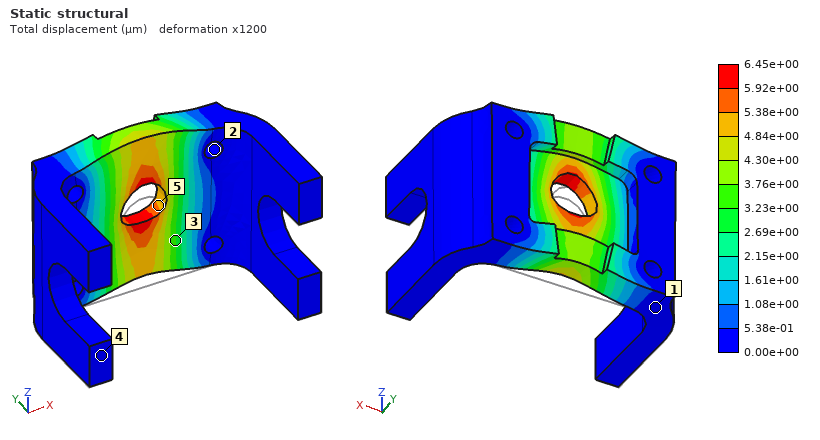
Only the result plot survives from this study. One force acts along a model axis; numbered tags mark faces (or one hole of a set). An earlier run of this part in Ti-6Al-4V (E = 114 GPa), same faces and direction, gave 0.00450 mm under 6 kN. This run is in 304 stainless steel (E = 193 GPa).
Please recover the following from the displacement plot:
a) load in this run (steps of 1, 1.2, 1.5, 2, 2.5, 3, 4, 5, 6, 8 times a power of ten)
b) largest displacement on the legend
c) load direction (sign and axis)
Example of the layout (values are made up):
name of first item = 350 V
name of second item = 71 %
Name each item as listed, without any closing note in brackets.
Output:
load in this run = 15 kN
largest displacement on the legend = 6.45e+00 µm
load direction = +Z
